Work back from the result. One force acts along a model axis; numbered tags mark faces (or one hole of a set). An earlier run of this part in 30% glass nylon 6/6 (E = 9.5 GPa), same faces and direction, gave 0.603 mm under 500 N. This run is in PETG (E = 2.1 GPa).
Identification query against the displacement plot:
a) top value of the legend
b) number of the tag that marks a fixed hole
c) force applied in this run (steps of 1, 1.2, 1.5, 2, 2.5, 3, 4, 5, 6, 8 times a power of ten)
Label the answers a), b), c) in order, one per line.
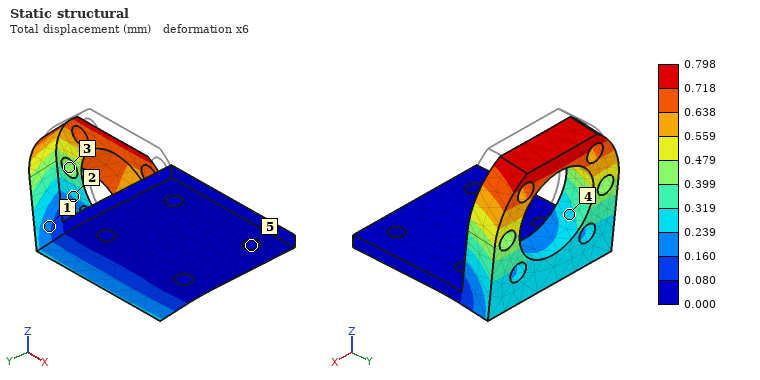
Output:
a) 0.798 mm
b) 5
c) 150 N
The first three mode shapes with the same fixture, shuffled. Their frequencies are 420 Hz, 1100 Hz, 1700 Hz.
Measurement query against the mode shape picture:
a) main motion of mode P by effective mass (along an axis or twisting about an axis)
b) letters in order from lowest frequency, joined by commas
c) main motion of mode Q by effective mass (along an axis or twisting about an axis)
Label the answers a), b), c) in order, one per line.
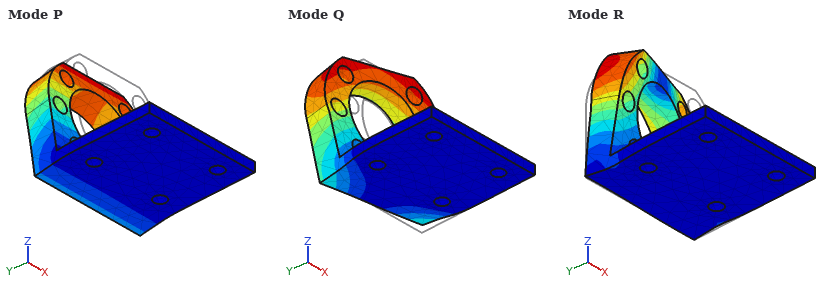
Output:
a) along Y
b) P, Q, R
c) along X
